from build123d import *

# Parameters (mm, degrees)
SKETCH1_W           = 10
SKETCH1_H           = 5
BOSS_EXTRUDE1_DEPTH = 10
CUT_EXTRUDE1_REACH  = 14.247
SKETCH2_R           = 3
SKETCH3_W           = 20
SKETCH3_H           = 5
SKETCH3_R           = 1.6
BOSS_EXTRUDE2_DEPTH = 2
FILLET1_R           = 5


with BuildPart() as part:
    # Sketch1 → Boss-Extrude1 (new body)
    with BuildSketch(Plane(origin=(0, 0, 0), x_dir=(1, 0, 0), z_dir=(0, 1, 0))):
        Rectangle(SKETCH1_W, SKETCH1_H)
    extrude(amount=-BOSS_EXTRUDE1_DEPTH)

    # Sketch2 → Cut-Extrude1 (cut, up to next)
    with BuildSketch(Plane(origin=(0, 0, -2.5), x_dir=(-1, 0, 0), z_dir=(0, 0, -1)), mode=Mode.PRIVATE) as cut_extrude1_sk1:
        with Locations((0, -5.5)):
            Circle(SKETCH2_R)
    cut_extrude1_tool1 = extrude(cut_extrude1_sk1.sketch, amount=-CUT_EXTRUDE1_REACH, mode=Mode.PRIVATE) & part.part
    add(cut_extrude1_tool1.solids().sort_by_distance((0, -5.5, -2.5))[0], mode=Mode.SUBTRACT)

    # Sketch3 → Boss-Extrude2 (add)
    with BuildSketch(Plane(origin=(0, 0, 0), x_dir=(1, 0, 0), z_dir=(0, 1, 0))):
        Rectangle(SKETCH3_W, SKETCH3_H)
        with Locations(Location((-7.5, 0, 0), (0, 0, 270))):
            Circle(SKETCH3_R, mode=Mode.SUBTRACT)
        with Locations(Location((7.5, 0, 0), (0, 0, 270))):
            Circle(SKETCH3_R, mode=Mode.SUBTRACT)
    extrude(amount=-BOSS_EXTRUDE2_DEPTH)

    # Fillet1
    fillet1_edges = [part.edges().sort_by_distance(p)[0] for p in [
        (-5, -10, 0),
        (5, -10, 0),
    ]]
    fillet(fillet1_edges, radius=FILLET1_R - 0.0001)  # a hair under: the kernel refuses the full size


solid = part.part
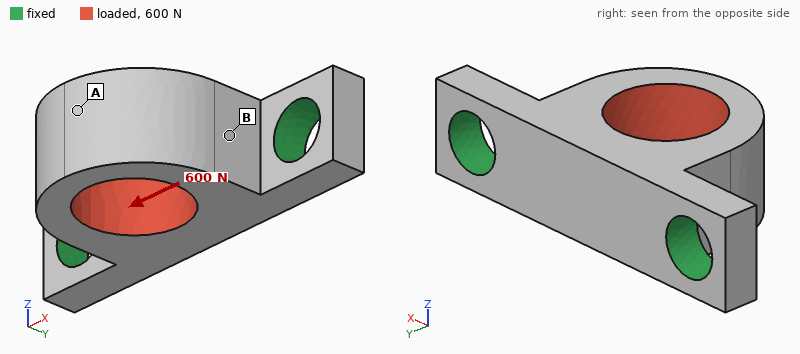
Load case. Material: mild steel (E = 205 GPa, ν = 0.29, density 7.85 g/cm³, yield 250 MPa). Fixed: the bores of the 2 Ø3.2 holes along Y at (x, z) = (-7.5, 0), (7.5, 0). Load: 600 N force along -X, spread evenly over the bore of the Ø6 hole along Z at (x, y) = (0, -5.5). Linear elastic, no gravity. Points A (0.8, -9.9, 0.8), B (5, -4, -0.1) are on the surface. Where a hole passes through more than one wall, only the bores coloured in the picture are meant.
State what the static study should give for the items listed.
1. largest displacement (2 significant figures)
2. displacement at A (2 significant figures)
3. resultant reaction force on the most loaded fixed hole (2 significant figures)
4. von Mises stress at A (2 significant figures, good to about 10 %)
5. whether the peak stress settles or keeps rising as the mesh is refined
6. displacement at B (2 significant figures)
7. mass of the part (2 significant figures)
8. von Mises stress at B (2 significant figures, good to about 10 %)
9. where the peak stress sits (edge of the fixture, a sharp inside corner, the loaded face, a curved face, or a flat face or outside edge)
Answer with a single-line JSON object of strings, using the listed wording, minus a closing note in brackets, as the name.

{"largest displacement": "6.9 µm", "displacement at A": "6.4 µm", "resultant reaction force on the most loaded fixed hole": "380 N", "von Mises stress at A": "20 MPa", "whether the peak stress settles or keeps rising as the mesh is refined": "keeps rising", "displacement at B": "2.5 µm", "mass of the part": "2.9 g", "von Mises stress at B": "63 MPa", "where the peak stress sits": "a sharp inside corner"}
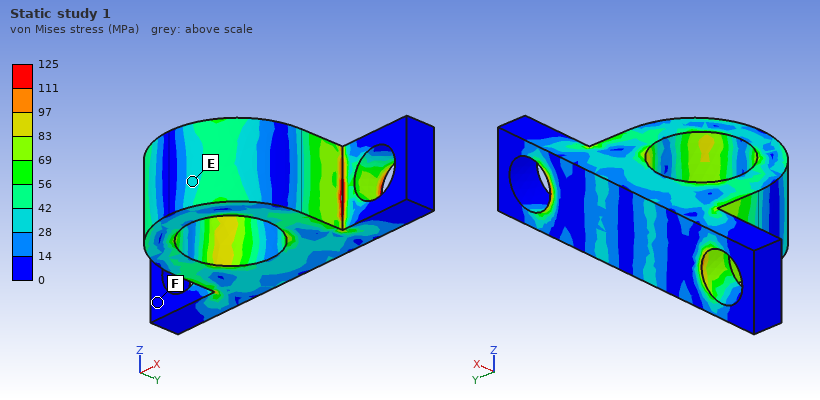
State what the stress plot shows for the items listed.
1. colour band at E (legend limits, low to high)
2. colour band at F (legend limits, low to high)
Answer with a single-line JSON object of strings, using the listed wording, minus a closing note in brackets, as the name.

{"colour band at E": "28 to 42 MPa", "colour band at F": "0 to 14 MPa"}
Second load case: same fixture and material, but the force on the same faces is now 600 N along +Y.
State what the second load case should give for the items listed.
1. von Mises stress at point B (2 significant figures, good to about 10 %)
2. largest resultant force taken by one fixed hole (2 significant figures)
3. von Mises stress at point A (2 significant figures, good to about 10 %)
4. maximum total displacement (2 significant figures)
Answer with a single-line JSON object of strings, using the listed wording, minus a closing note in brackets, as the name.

{"von Mises stress at point B": "42 MPa", "largest resultant force taken by one fixed hole": "320 N", "von Mises stress at point A": "14 MPa", "maximum total displacement": "2.5 µm"}
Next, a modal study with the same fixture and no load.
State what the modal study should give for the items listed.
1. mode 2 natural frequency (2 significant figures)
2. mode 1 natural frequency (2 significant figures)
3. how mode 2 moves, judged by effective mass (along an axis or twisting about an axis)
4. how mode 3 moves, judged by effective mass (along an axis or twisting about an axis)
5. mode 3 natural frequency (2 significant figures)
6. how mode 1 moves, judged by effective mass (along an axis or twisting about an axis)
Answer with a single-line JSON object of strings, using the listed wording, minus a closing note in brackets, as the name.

{"mode 2 natural frequency": "42 kHz", "mode 1 natural frequency": "22 kHz", "how mode 2 moves, judged by effective mass": "along X", "how mode 3 moves, judged by effective mass": "along Y", "mode 3 natural frequency": "56 kHz", "how mode 1 moves, judged by effective mass": "along Z"}
